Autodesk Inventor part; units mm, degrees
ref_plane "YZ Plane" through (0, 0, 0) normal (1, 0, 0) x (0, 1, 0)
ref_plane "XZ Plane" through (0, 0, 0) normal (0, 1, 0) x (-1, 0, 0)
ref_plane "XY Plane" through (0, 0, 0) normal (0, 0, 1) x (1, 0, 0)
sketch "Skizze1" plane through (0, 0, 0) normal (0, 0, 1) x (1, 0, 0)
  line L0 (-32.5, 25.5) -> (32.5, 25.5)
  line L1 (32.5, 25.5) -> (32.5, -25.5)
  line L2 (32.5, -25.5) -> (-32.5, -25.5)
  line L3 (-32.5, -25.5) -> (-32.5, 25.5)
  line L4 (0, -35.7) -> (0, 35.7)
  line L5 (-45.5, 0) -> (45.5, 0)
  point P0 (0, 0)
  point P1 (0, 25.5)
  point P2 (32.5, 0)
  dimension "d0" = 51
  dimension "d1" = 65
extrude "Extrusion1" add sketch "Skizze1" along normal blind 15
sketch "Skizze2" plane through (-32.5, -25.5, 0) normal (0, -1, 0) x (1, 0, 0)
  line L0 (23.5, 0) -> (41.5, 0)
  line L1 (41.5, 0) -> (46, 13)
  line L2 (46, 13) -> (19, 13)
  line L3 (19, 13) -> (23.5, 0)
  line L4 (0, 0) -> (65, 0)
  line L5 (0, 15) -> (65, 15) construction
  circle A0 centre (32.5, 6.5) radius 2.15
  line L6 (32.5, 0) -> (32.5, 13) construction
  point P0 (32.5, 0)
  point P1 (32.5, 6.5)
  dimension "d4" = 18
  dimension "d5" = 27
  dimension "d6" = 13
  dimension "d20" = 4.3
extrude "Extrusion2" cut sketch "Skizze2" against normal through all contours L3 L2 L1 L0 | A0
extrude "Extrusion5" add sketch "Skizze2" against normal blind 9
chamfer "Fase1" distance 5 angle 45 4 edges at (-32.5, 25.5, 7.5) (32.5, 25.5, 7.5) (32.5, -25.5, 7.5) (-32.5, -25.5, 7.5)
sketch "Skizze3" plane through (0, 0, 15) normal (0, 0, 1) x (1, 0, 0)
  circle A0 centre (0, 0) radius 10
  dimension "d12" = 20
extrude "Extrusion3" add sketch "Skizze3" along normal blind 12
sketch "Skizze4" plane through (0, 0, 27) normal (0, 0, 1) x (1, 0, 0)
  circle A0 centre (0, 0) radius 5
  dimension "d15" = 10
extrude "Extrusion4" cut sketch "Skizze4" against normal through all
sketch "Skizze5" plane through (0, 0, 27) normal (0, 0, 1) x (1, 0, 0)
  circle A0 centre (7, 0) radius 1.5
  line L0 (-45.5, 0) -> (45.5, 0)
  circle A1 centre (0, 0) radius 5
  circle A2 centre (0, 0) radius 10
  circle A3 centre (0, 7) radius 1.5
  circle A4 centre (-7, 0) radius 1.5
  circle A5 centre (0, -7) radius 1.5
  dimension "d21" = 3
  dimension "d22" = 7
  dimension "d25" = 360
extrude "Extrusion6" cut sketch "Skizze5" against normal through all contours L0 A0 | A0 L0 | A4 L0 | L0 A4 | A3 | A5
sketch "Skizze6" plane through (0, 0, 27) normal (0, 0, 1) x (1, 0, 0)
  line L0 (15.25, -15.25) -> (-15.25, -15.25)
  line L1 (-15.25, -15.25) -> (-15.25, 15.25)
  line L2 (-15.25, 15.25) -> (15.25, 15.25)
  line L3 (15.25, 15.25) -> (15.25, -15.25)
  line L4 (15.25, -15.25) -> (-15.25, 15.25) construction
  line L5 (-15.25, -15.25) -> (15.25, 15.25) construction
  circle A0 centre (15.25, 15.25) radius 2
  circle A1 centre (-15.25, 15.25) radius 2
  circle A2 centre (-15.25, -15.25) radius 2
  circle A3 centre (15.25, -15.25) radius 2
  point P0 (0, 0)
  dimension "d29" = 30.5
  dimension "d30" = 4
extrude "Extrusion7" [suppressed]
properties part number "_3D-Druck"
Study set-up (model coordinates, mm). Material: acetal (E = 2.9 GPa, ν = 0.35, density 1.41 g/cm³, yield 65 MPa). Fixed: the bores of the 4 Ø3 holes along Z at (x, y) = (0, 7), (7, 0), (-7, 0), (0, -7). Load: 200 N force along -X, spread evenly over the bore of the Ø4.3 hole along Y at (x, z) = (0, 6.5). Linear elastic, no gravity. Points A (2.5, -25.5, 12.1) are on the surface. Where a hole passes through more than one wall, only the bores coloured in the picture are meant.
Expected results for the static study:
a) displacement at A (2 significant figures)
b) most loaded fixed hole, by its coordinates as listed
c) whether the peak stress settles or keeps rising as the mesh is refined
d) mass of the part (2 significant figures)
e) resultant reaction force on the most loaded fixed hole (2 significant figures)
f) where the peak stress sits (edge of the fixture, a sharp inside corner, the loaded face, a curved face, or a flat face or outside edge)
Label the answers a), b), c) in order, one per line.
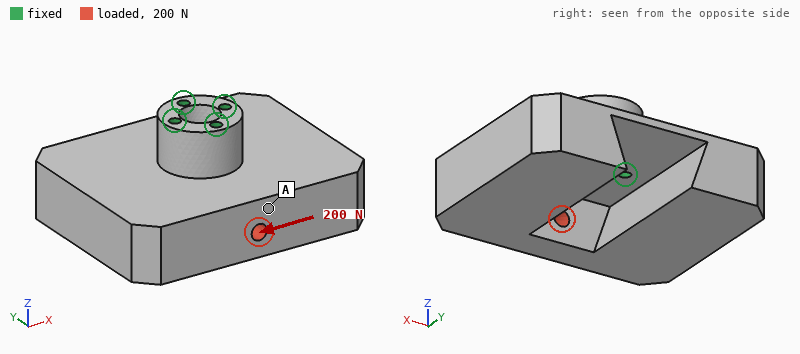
a) 0.086 mm
b) (0, -7)
c) keeps rising
d) 55 g
e) 200 N
f) edge of the fixture
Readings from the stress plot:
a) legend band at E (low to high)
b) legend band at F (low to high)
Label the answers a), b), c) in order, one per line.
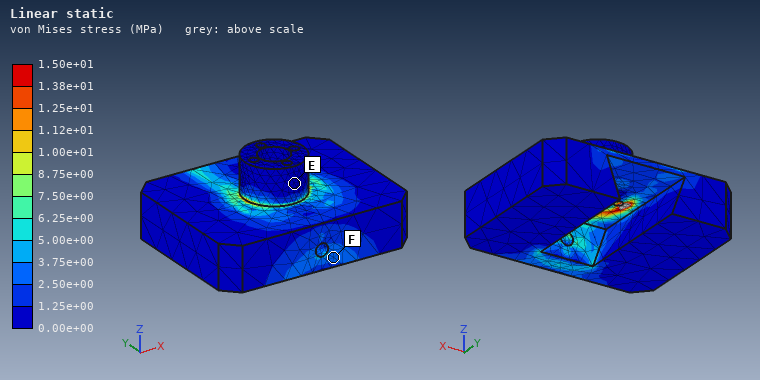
a) 0.00e+00 to 1.25e+00 MPa
b) 2.50e+00 to 3.75e+00 MPa
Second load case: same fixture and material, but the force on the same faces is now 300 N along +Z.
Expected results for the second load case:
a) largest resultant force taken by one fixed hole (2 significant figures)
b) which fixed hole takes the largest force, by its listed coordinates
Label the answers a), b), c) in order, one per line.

a) 290 N
b) (0, -7)
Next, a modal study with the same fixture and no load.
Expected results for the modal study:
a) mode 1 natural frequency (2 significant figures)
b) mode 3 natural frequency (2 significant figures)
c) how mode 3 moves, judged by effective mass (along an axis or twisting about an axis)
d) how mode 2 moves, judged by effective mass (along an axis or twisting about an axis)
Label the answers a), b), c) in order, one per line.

a) 450 Hz
b) 1100 Hz
c) along Z
d) along Y
